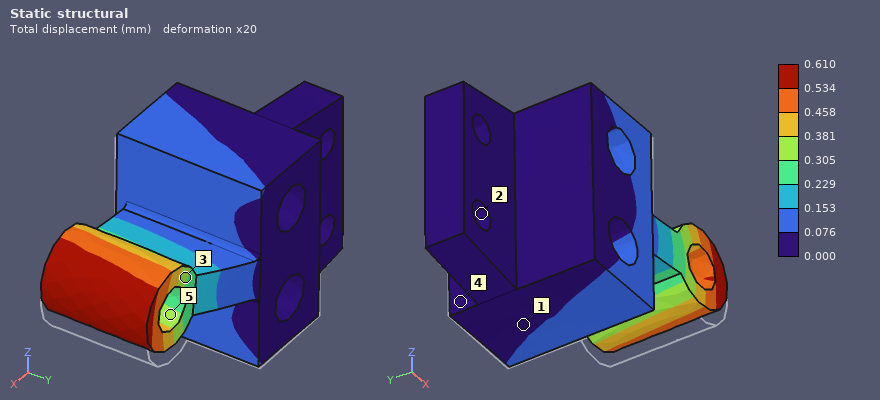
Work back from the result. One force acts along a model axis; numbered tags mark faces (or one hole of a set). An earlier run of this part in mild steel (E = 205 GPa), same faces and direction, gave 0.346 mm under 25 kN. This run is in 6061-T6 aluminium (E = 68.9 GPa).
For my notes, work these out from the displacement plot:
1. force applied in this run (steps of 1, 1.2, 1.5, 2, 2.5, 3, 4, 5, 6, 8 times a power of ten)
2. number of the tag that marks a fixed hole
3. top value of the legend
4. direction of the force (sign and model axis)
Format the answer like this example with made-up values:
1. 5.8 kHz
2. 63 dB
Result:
1. 15 kN
2. 2
3. 0.610 mm
4. +Z
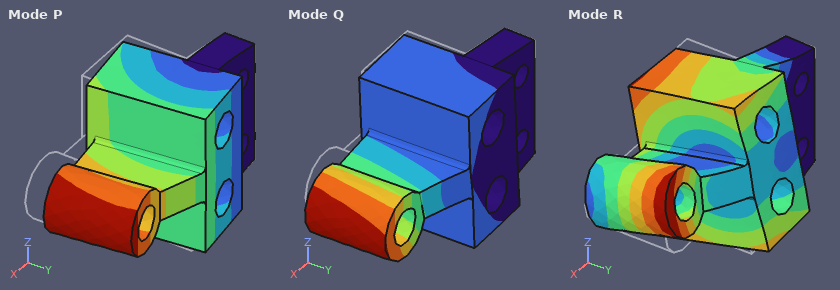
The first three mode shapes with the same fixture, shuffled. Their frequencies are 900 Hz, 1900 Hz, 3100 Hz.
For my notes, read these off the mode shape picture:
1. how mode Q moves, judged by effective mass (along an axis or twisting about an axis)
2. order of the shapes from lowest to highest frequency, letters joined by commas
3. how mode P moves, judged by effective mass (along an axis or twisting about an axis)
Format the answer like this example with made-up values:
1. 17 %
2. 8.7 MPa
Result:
1. along Z
2. P, Q, R
3. along Y
